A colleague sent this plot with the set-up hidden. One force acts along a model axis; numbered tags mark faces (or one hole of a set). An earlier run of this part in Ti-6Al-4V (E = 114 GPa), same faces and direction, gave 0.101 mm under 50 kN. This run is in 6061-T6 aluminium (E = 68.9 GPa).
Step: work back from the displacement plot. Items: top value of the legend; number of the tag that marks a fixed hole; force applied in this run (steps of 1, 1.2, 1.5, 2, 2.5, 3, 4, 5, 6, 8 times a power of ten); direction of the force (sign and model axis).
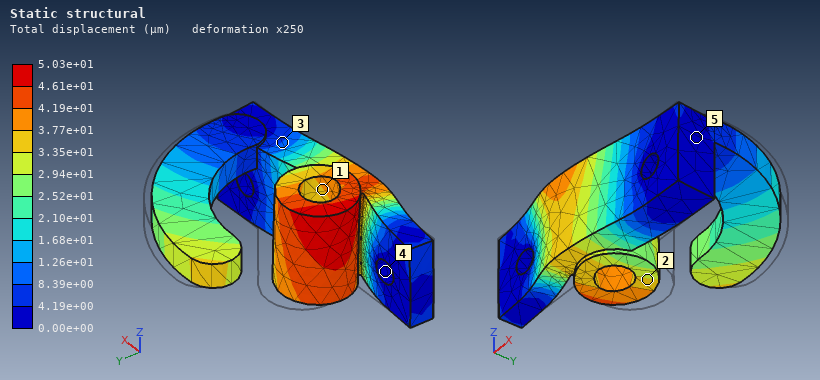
5.03e+01 µm
4
15 kN
-Y
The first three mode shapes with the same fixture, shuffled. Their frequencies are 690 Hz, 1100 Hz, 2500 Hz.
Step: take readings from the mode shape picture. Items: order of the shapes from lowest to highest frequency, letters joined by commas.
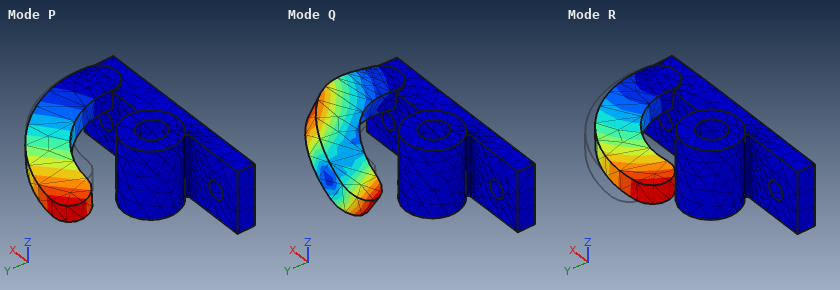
P, R, Q
